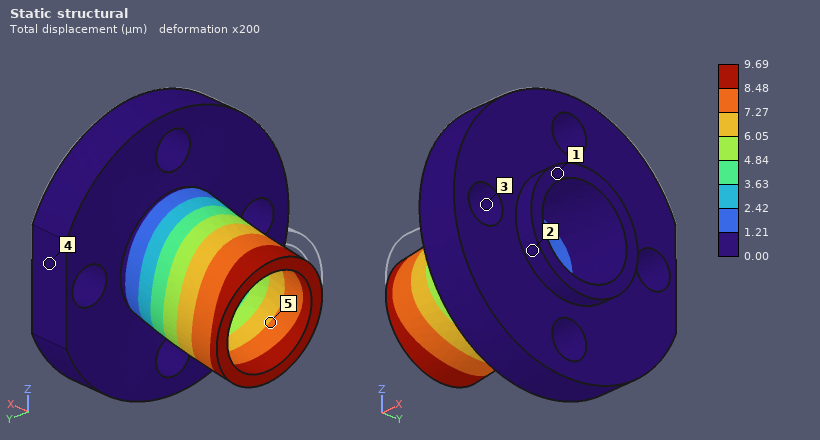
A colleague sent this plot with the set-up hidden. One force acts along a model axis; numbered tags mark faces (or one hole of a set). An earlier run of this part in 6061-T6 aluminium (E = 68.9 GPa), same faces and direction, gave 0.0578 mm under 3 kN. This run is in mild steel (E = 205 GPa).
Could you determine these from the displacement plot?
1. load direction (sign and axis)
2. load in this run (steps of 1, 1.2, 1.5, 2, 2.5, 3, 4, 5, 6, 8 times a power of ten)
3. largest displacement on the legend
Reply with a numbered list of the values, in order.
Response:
1. -Z
2. 1.5 kN
3. 9.69 µm
